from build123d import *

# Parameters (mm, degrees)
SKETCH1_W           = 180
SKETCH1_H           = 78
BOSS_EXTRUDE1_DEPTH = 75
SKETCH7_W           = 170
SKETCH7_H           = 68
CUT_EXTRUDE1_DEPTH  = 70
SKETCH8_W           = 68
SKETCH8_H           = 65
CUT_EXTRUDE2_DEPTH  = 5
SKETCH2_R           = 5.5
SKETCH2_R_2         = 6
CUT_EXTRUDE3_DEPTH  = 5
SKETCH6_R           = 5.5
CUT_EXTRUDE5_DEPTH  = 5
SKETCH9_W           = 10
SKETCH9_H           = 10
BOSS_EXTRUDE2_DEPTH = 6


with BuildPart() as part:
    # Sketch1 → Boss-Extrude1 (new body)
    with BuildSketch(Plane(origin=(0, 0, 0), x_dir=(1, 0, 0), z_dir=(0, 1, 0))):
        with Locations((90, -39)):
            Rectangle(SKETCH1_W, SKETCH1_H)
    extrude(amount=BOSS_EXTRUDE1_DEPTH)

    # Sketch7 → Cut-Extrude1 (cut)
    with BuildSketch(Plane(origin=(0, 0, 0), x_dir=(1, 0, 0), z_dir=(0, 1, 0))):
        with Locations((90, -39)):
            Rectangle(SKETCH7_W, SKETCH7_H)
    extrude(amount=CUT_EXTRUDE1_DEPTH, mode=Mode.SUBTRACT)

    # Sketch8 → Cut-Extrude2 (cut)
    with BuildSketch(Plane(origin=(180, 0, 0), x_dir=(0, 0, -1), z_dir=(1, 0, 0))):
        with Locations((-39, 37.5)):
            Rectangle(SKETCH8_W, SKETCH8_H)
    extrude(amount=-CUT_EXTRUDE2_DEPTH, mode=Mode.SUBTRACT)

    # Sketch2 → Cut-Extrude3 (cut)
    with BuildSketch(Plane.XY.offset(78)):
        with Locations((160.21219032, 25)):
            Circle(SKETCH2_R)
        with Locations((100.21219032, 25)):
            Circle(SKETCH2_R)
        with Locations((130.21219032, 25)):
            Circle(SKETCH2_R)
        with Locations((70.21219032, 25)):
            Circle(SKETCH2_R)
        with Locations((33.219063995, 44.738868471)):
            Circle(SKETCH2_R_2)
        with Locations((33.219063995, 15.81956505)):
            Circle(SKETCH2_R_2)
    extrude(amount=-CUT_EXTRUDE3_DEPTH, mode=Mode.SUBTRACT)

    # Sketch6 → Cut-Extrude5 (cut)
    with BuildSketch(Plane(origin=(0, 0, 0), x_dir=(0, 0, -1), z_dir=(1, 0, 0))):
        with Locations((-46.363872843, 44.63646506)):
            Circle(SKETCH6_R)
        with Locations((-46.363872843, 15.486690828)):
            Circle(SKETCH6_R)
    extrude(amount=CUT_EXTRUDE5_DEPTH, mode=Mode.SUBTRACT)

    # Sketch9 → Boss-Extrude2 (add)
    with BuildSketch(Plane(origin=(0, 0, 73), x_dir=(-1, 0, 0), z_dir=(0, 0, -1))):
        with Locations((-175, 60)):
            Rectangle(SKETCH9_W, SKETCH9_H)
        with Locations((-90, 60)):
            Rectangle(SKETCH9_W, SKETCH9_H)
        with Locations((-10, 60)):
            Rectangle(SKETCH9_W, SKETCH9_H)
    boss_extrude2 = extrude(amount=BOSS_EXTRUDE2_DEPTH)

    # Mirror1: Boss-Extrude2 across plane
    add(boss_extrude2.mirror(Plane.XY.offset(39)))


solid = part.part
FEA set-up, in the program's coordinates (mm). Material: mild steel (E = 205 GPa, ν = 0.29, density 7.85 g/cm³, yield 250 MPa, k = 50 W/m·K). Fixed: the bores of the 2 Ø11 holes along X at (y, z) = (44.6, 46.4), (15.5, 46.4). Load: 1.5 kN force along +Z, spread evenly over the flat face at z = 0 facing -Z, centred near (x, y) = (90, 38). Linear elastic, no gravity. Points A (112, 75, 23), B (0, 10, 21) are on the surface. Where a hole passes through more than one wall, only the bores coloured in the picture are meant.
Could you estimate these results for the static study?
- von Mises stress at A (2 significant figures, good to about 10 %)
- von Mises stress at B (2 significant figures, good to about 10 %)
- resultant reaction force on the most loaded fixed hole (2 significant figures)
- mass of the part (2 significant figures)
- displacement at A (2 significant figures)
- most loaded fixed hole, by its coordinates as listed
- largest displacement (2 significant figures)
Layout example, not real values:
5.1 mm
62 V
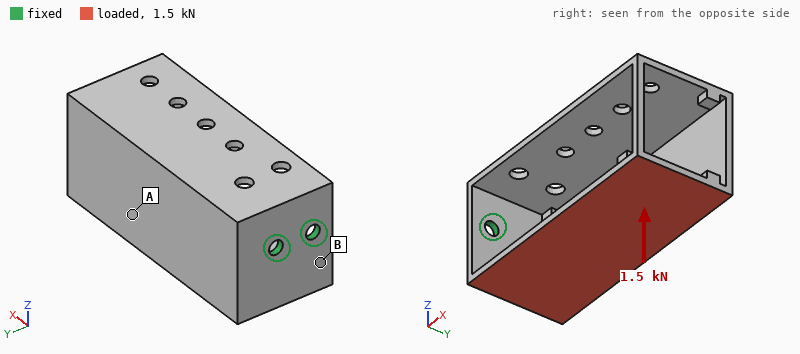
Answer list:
28 MPa
96 MPa
950 N
1.7 kg
0.67 mm
(44.6, 46.4)
1.6 mm
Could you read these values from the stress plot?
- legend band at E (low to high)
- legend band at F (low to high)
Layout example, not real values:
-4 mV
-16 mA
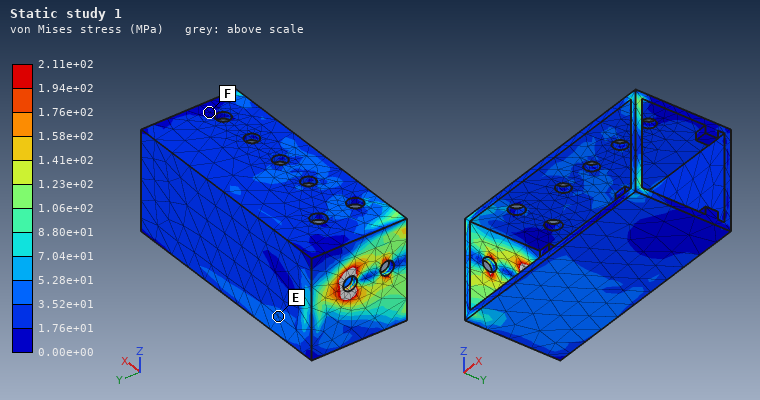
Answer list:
3.52e+01 to 5.28e+01 MPa
0.00e+00 to 1.76e+01 MPa
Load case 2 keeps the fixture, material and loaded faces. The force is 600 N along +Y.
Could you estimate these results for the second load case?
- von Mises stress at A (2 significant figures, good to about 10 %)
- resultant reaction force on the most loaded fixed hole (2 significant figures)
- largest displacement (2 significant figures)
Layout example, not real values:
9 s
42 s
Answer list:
9.0 MPa
1.4 kN
0.35 mm
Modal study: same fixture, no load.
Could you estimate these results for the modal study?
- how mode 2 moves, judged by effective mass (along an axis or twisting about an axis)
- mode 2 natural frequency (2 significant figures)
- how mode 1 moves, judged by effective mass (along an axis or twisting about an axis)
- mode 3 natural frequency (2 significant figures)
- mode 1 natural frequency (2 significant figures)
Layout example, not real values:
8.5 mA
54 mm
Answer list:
along Y
260 Hz
along Z
600 Hz
160 Hz
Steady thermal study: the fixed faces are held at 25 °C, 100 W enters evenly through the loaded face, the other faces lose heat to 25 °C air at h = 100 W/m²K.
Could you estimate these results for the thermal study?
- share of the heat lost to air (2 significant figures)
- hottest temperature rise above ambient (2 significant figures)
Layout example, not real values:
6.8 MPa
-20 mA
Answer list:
93 %
47 K
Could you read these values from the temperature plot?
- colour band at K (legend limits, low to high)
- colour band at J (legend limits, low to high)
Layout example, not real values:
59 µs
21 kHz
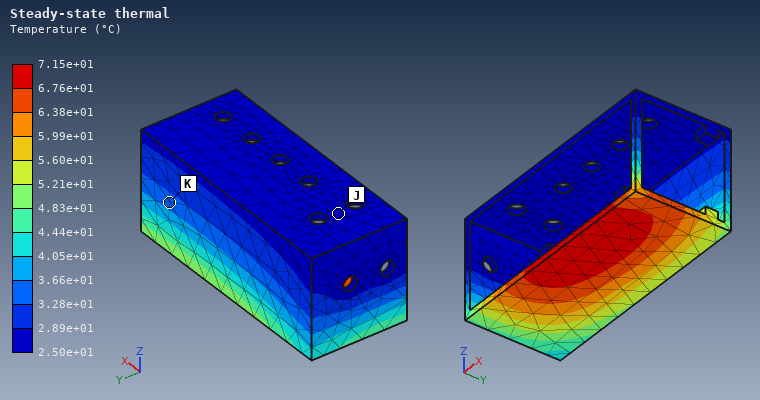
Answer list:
3.28e+01 to 3.66e+01 °C
2.50e+01 to 2.89e+01 °C
